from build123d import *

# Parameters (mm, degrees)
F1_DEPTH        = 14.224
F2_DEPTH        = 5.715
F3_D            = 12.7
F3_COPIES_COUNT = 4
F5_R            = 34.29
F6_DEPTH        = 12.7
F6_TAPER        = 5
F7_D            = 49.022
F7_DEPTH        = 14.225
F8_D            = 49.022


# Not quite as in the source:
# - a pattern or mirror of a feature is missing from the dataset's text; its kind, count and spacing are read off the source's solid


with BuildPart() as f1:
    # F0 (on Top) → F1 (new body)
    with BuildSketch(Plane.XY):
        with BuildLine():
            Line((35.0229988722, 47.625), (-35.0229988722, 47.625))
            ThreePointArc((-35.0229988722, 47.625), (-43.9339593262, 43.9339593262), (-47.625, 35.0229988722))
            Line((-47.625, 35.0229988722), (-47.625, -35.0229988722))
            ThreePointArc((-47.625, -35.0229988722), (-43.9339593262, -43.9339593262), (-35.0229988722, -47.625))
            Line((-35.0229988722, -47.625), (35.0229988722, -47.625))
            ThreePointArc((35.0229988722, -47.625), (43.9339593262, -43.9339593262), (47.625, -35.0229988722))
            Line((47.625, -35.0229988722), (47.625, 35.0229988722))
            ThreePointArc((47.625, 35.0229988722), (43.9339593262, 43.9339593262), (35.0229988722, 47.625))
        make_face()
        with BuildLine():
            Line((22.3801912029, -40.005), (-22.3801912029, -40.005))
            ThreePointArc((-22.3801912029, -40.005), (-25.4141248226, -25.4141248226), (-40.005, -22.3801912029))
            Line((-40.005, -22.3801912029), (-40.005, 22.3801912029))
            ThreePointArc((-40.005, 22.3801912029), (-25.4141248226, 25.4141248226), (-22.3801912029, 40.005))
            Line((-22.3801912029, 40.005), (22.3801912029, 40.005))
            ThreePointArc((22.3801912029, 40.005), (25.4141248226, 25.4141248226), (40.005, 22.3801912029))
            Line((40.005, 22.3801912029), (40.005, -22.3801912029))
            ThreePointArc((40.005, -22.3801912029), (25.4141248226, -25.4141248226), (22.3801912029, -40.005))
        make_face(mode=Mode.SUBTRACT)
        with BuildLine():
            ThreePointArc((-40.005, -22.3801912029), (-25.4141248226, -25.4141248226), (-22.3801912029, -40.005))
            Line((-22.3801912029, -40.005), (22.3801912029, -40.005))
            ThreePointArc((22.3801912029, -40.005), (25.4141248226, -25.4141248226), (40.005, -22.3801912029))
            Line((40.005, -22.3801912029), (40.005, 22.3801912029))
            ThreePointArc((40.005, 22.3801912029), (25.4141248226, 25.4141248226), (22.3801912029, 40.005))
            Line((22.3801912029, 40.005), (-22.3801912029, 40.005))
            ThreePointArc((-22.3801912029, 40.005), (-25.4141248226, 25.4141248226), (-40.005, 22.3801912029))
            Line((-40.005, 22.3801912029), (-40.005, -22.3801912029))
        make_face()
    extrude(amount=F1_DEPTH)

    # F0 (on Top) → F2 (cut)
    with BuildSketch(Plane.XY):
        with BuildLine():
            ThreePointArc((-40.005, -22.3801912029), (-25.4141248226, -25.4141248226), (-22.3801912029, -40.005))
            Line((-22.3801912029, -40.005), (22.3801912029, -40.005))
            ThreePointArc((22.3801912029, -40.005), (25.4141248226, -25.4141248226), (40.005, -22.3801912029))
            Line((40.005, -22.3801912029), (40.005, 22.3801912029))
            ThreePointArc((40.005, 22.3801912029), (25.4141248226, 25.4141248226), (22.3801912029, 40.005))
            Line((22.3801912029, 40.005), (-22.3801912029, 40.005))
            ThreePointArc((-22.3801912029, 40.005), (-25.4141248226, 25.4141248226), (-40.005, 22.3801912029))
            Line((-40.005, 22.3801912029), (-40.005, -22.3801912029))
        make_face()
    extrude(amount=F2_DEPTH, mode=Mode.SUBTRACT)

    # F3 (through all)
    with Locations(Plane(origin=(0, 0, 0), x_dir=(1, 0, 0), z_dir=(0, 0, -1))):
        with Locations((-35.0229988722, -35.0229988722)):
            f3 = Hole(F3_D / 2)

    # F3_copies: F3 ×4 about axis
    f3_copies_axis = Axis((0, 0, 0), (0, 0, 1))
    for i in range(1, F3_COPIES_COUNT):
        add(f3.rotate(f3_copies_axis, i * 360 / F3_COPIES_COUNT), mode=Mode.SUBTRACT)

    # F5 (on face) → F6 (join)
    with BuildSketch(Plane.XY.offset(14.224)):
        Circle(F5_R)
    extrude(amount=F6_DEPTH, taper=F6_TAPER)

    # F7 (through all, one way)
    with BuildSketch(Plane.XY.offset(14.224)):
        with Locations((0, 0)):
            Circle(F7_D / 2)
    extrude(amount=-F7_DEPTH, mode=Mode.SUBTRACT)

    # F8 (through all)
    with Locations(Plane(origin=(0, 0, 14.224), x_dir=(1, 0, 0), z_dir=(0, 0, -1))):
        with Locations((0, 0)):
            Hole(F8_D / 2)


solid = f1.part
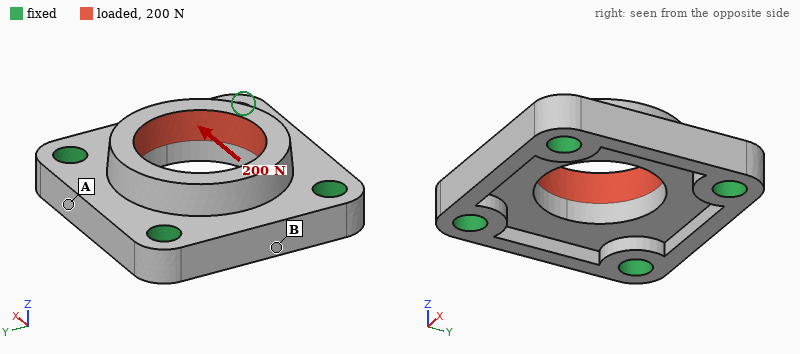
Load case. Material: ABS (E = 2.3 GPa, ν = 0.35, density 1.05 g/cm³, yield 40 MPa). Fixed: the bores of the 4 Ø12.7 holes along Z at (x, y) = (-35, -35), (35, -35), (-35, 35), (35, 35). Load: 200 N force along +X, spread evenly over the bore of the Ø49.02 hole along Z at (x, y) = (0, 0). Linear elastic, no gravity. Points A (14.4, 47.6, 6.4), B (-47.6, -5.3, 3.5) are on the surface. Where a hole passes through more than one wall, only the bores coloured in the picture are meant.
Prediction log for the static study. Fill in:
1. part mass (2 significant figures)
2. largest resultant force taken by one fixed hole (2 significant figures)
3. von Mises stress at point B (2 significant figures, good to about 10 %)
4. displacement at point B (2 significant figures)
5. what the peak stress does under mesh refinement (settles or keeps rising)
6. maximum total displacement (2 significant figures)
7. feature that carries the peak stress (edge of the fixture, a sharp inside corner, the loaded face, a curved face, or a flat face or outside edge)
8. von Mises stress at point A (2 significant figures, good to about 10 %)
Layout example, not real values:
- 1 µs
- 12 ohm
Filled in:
- 100 g
- 54 N
- 0.15 MPa
- 3.0 µm
- keeps rising
- 8.8 µm
- edge of the fixture
- 0.058 MPa
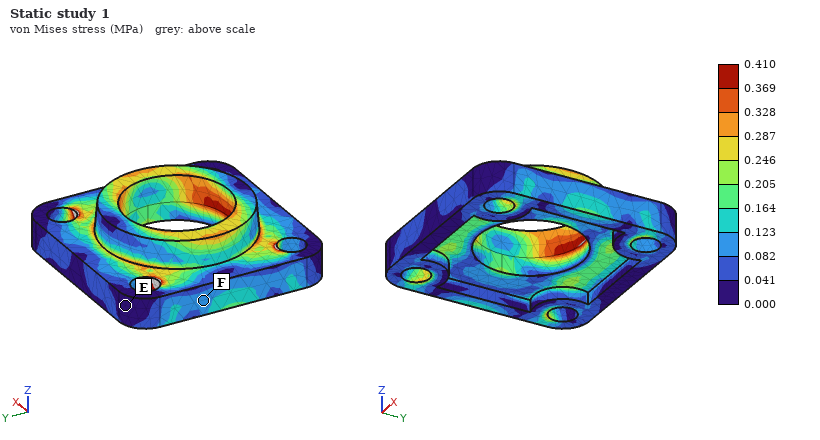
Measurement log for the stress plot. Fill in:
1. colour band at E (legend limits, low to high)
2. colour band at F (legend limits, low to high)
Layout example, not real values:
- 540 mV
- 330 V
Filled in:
- 0.000 to 0.041 MPa
- 0.082 to 0.123 MPa
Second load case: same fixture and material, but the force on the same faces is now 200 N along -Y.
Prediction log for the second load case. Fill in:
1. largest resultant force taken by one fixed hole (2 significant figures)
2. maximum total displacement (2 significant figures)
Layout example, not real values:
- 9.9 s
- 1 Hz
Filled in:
- 54 N
- 8.8 µm
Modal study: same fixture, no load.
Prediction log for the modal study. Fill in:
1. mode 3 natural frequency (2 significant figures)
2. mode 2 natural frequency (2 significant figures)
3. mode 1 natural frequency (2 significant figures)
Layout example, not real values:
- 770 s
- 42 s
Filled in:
- 4300 Hz
- 4000 Hz
- 4000 Hz
